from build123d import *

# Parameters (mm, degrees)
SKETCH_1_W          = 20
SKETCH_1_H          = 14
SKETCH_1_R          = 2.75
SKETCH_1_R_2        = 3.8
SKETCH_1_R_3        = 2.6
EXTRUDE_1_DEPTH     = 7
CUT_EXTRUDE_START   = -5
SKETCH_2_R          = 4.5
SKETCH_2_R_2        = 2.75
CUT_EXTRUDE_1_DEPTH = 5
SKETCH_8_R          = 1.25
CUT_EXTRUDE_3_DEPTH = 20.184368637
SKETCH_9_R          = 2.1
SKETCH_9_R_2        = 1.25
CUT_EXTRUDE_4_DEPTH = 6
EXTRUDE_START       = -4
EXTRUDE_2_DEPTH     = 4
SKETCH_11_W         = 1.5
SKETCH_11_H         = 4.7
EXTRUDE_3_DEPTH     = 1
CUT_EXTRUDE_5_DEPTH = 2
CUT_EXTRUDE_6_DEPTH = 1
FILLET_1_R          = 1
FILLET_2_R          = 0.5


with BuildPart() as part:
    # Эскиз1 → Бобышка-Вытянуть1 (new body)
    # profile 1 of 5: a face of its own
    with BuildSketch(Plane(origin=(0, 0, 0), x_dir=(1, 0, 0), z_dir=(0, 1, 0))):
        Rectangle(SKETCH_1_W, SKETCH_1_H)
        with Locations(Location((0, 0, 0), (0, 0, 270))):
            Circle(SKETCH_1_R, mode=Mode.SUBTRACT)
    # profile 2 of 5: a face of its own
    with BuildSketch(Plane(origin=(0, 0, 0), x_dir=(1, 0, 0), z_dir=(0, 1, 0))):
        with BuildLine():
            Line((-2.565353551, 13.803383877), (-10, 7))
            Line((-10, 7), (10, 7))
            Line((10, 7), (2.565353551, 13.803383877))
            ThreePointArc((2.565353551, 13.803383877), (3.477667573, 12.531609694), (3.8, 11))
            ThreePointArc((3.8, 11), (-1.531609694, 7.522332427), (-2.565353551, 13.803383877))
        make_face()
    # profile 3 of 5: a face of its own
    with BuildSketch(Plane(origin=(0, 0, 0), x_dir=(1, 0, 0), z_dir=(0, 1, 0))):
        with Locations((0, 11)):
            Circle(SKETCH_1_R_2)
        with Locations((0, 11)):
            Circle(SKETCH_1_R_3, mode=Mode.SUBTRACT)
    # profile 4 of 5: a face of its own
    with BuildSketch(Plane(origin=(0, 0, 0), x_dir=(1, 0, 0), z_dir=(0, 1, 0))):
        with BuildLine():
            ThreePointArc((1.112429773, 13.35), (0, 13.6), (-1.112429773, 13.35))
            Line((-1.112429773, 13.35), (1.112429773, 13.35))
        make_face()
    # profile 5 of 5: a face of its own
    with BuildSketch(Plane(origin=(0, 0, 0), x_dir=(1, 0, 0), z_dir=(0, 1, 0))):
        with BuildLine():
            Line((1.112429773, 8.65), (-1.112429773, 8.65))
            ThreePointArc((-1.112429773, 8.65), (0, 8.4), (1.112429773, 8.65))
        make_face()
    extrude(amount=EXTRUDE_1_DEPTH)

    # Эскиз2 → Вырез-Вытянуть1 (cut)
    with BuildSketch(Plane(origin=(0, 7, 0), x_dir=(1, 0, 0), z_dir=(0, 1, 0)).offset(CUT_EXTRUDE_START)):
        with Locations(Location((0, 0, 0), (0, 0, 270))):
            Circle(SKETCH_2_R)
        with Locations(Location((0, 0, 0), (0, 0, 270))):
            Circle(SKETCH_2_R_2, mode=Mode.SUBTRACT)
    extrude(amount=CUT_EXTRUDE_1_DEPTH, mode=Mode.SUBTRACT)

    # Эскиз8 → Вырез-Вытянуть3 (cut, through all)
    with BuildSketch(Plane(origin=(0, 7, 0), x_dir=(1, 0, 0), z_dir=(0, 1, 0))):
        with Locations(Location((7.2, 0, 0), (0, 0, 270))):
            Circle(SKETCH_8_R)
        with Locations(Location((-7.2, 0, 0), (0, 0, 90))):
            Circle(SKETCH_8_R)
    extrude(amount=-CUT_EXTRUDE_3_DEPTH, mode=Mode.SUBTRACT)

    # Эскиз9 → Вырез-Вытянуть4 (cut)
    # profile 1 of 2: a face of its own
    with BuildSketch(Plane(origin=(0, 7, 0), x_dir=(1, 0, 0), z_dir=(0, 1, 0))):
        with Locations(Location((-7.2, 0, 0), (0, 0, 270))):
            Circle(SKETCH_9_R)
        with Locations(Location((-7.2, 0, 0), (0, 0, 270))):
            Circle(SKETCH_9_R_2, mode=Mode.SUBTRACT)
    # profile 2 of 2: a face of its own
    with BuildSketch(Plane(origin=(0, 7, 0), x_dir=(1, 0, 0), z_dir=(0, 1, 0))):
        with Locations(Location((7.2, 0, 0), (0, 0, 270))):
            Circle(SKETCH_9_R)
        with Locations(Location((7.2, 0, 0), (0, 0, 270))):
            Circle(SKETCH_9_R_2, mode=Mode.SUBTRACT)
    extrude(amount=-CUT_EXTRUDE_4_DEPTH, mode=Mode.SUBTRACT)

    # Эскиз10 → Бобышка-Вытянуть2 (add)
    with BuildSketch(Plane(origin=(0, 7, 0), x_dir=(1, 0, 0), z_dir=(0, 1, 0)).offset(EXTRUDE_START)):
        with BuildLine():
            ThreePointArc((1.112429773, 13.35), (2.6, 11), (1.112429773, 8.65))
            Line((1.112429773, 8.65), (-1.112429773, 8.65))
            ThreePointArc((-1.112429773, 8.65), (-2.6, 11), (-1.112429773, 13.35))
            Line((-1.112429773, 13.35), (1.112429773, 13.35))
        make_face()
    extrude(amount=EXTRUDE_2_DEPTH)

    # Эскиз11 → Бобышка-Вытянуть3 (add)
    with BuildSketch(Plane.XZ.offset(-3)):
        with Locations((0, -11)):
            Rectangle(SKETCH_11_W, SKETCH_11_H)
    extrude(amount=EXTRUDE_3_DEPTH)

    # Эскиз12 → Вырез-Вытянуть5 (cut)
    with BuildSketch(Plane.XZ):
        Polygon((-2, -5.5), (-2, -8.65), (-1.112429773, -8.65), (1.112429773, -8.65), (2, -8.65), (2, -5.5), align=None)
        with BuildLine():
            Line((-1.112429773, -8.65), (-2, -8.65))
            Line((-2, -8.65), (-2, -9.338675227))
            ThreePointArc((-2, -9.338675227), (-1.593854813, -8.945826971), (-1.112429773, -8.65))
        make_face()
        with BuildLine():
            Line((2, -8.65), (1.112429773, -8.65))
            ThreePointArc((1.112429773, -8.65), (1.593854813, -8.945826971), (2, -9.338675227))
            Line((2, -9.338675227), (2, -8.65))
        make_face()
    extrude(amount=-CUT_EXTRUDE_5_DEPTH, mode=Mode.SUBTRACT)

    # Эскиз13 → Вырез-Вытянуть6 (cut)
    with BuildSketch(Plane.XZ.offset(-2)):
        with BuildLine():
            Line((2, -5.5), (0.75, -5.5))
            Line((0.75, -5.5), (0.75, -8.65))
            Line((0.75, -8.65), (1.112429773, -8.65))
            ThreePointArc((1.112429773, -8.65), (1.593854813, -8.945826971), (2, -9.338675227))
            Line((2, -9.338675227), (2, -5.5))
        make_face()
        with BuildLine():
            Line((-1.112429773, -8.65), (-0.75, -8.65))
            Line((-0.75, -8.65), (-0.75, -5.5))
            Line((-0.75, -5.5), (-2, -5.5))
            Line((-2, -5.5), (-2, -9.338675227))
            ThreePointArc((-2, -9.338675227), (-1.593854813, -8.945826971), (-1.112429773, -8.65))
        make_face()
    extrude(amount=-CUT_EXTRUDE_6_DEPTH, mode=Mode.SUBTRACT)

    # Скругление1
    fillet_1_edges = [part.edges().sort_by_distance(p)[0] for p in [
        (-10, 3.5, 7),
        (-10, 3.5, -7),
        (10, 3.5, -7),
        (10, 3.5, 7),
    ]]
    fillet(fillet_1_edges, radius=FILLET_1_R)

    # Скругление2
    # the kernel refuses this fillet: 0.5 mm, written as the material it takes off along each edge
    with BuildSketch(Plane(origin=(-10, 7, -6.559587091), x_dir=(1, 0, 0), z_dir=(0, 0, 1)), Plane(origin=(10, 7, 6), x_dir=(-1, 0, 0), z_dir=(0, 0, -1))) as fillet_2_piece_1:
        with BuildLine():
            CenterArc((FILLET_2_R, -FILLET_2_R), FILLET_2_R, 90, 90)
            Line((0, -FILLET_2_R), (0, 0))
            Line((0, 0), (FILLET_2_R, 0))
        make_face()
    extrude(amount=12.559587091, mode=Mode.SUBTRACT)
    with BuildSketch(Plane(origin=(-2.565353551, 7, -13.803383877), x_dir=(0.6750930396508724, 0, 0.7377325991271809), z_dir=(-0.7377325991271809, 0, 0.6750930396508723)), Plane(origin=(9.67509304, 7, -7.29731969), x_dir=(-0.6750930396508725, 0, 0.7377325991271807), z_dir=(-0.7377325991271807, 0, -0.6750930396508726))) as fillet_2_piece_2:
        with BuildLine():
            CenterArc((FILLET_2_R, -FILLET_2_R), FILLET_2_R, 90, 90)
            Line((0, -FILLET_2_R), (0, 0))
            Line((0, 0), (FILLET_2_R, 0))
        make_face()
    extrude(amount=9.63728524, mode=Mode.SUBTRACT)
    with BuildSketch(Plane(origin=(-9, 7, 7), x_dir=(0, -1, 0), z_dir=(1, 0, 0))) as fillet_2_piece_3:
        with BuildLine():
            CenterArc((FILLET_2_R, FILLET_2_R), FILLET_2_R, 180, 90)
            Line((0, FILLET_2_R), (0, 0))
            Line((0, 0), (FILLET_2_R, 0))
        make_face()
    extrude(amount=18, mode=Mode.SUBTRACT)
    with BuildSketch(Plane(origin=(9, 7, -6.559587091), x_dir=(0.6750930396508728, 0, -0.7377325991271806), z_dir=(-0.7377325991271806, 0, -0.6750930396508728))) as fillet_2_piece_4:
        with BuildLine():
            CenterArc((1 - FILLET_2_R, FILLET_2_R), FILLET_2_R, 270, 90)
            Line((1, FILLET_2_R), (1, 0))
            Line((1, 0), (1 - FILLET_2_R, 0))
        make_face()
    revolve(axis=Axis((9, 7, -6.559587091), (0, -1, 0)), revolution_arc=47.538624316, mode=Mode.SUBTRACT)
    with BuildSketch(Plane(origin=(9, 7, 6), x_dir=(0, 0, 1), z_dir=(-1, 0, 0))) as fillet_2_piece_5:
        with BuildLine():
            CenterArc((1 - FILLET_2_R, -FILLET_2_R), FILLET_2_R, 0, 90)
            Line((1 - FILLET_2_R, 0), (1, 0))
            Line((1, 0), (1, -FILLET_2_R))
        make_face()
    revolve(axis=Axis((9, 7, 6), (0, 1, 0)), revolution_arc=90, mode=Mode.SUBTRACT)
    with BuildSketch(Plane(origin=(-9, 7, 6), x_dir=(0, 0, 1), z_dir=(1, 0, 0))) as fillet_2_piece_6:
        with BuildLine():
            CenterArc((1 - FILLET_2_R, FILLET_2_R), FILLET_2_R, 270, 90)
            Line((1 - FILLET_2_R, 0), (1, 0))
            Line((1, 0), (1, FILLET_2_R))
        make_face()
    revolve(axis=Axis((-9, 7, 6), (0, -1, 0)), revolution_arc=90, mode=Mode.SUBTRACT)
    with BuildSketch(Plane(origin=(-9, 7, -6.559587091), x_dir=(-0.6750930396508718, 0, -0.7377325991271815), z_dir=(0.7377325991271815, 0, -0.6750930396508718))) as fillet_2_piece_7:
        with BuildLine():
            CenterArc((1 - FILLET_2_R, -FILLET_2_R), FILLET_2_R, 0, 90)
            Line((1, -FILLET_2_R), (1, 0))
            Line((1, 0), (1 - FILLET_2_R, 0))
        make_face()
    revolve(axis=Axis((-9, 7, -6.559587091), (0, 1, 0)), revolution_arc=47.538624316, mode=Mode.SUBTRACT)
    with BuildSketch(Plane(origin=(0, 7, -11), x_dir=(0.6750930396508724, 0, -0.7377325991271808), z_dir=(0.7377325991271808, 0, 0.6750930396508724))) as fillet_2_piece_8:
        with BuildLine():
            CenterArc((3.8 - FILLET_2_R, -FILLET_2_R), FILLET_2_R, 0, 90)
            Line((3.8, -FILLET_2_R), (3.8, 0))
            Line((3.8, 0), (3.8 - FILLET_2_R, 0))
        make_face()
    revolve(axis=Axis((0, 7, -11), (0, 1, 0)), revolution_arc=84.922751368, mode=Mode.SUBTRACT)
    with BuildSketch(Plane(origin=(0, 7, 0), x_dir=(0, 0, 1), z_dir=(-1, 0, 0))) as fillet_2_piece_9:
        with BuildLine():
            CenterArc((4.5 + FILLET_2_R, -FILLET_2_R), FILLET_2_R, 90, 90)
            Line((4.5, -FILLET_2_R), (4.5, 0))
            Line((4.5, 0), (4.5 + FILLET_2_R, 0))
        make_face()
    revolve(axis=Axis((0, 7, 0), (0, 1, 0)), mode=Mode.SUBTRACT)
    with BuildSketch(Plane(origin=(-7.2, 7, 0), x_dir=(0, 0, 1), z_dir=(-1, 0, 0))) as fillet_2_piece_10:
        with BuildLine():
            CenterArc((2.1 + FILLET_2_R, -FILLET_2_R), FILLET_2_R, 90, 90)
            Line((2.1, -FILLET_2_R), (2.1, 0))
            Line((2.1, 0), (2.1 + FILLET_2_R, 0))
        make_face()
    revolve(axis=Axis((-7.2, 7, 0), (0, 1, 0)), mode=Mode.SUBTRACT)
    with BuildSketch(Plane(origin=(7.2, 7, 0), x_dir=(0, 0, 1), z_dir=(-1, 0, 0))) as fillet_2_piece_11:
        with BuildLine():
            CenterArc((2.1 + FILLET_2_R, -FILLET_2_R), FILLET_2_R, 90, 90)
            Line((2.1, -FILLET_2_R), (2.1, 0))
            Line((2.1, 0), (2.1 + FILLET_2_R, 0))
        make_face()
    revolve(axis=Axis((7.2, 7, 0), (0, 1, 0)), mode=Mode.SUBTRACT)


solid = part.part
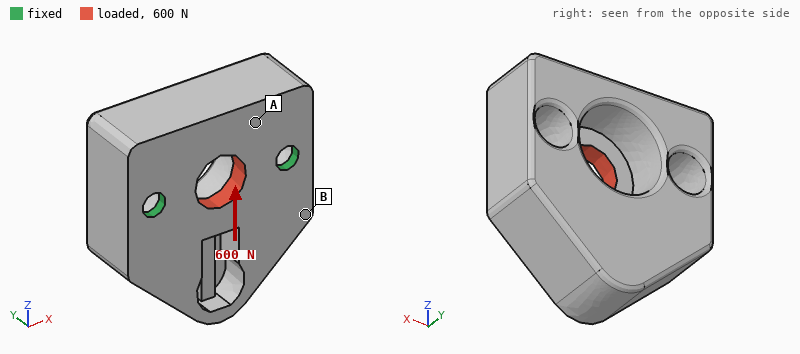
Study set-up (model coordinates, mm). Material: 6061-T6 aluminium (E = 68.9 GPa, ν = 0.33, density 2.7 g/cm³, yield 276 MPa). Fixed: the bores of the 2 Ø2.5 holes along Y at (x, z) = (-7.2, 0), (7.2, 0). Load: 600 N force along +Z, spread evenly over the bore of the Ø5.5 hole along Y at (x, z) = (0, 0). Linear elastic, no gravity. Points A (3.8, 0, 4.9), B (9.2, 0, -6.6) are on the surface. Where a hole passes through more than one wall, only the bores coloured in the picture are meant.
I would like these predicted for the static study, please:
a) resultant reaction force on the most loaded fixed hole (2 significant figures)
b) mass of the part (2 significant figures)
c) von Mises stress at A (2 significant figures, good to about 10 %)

300 N
5.2 g
17 MPa
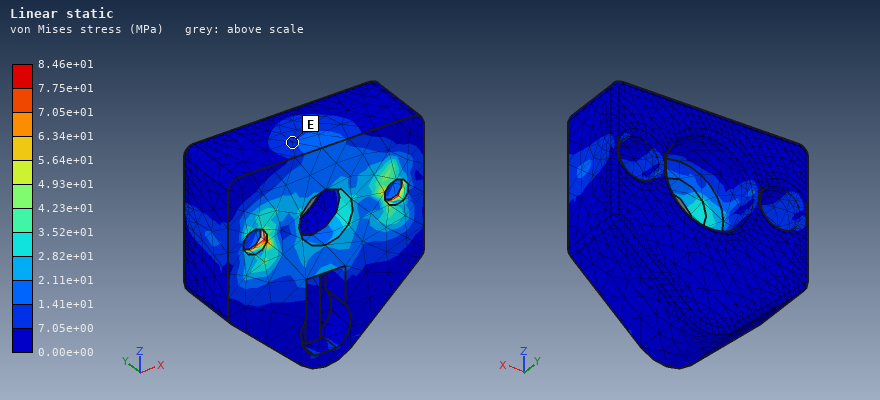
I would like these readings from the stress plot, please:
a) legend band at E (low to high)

7.05e+00 to 1.41e+01 MPa
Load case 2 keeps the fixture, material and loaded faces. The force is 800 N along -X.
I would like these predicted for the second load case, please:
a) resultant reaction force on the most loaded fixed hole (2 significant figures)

400 N
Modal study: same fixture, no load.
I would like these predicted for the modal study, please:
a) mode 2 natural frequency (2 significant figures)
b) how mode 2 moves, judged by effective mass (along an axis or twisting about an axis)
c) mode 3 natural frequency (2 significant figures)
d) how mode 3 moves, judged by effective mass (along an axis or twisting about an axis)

26 kHz
along X
28 kHz
along Y
